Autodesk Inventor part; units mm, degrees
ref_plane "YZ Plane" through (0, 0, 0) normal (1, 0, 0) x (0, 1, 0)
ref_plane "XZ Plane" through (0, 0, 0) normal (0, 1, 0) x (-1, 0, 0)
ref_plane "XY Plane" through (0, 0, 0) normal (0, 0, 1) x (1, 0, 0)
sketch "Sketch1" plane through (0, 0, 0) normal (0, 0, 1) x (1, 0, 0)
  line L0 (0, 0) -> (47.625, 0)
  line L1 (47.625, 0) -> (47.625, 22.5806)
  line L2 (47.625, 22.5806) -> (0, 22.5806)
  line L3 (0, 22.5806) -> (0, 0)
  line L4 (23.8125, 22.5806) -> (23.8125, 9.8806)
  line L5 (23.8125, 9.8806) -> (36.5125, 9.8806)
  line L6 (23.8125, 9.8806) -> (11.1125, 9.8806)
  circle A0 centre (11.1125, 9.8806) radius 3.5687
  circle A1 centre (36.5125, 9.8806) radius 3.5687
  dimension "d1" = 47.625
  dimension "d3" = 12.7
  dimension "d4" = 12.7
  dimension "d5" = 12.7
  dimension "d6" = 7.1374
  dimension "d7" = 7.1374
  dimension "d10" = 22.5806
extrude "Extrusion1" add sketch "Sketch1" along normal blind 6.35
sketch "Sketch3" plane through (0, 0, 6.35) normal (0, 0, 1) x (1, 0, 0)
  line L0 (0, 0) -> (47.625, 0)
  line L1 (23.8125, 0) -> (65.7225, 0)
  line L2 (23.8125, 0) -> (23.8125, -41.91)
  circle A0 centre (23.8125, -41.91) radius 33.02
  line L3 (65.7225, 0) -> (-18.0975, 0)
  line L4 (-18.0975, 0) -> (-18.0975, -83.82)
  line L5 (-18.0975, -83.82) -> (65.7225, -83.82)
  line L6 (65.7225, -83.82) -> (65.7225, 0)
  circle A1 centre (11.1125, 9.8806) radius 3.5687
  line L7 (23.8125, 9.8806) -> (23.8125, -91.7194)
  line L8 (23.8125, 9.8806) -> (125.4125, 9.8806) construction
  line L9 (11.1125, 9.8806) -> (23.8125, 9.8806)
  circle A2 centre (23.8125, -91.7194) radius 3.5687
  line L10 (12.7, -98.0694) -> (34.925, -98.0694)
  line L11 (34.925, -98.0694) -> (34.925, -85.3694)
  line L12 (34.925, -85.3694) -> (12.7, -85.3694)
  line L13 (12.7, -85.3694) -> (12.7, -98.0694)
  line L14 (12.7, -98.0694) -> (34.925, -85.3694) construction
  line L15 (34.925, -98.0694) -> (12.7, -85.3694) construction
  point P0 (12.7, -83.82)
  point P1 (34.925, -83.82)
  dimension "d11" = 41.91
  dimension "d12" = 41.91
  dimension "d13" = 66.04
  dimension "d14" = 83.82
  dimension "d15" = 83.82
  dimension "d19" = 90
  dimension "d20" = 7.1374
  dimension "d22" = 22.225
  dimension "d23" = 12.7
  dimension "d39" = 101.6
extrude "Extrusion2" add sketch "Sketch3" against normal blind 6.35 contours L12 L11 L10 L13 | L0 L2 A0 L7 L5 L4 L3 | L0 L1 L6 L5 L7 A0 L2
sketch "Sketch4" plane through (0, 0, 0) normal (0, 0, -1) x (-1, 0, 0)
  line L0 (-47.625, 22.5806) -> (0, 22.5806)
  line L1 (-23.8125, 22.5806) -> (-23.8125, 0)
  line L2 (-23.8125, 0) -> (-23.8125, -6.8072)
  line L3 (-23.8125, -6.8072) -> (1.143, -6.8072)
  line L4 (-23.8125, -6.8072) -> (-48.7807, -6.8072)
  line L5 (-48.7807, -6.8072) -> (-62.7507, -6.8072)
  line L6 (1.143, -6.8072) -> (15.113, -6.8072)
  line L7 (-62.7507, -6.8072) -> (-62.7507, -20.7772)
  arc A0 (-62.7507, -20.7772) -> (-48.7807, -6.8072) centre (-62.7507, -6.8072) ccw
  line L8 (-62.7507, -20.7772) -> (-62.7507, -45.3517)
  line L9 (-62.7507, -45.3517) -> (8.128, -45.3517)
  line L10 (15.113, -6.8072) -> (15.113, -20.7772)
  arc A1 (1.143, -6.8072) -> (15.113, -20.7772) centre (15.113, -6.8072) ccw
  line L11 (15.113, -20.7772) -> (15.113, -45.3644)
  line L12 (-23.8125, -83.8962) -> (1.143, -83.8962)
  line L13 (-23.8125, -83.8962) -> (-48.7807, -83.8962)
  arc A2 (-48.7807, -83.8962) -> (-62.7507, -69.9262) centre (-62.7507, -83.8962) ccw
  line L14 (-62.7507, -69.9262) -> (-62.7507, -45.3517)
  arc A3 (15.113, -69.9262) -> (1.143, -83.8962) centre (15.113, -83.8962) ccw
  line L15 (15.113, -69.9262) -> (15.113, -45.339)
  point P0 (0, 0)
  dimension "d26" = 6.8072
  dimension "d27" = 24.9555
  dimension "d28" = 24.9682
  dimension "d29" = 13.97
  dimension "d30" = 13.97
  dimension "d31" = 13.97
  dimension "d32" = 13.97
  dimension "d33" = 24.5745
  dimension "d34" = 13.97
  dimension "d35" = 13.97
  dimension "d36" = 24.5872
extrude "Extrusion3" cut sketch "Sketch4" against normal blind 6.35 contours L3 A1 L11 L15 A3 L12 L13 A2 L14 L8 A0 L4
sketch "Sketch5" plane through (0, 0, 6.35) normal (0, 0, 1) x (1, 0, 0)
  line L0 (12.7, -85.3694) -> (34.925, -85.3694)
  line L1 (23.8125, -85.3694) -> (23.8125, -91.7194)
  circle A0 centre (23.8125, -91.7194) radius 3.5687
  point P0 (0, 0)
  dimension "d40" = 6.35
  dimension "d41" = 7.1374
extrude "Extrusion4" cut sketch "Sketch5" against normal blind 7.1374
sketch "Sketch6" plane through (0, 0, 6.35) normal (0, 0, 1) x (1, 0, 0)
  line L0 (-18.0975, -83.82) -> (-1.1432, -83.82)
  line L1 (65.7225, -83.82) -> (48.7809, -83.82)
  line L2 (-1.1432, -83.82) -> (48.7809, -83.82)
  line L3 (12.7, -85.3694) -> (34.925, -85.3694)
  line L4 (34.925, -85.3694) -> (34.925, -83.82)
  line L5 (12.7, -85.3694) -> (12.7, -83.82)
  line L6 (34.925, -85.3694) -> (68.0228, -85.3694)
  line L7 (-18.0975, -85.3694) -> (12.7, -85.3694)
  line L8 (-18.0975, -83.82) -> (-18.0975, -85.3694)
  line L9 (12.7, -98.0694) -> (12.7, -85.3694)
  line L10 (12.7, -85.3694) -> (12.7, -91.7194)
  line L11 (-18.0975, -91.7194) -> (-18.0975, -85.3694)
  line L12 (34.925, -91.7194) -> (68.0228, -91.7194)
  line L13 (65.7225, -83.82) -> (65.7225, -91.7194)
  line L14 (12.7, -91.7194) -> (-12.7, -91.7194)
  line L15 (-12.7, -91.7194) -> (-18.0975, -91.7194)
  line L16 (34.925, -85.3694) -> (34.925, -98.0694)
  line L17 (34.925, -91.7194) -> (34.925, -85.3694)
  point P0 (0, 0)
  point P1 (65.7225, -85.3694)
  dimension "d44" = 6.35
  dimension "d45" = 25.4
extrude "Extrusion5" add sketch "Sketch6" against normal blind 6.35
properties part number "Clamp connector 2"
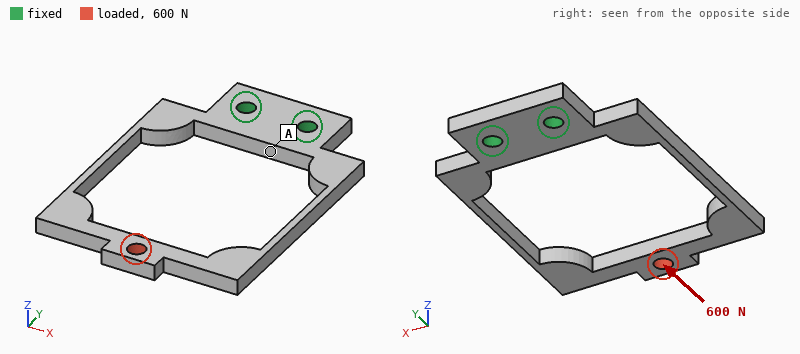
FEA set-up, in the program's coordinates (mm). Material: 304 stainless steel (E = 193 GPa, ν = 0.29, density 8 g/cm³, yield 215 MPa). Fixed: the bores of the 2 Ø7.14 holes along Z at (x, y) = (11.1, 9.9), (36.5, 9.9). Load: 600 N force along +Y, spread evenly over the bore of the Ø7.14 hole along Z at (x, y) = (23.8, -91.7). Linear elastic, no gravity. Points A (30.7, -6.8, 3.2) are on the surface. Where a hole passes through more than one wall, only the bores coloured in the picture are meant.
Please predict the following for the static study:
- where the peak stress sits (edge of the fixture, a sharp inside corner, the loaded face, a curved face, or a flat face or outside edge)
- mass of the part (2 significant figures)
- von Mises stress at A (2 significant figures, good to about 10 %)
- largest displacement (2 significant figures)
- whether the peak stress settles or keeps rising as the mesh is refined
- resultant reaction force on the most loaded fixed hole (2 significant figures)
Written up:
a sharp inside corner
170 g
12 MPa
0.11 mm
keeps rising
480 N
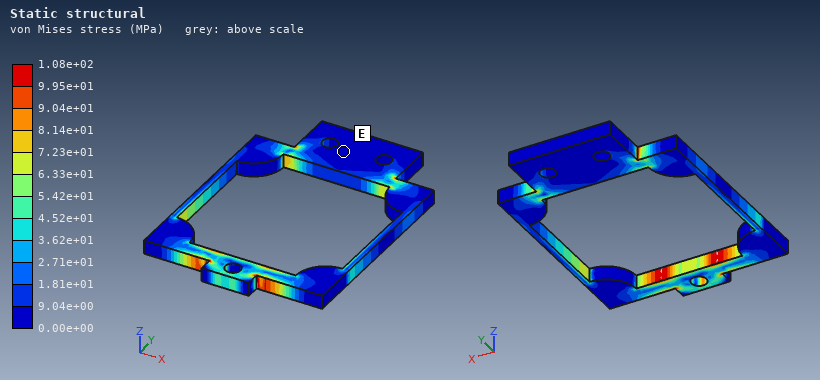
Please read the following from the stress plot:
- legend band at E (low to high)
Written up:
0.00e+00 to 9.04e+00 MPa
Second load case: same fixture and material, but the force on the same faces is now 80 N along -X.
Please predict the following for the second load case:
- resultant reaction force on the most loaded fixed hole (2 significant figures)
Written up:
240 N
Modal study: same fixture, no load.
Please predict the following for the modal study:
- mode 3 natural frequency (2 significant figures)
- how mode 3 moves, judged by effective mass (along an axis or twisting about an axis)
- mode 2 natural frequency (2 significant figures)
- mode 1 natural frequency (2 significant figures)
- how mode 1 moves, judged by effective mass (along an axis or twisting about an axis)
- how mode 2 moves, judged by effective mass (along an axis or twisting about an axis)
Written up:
650 Hz
twisting about Y
370 Hz
240 Hz
along Z
along X
